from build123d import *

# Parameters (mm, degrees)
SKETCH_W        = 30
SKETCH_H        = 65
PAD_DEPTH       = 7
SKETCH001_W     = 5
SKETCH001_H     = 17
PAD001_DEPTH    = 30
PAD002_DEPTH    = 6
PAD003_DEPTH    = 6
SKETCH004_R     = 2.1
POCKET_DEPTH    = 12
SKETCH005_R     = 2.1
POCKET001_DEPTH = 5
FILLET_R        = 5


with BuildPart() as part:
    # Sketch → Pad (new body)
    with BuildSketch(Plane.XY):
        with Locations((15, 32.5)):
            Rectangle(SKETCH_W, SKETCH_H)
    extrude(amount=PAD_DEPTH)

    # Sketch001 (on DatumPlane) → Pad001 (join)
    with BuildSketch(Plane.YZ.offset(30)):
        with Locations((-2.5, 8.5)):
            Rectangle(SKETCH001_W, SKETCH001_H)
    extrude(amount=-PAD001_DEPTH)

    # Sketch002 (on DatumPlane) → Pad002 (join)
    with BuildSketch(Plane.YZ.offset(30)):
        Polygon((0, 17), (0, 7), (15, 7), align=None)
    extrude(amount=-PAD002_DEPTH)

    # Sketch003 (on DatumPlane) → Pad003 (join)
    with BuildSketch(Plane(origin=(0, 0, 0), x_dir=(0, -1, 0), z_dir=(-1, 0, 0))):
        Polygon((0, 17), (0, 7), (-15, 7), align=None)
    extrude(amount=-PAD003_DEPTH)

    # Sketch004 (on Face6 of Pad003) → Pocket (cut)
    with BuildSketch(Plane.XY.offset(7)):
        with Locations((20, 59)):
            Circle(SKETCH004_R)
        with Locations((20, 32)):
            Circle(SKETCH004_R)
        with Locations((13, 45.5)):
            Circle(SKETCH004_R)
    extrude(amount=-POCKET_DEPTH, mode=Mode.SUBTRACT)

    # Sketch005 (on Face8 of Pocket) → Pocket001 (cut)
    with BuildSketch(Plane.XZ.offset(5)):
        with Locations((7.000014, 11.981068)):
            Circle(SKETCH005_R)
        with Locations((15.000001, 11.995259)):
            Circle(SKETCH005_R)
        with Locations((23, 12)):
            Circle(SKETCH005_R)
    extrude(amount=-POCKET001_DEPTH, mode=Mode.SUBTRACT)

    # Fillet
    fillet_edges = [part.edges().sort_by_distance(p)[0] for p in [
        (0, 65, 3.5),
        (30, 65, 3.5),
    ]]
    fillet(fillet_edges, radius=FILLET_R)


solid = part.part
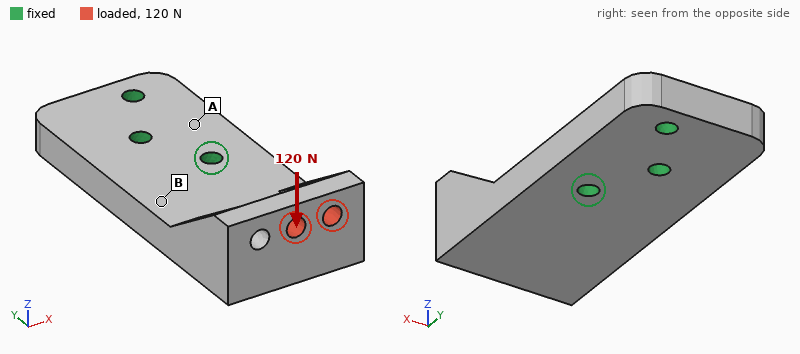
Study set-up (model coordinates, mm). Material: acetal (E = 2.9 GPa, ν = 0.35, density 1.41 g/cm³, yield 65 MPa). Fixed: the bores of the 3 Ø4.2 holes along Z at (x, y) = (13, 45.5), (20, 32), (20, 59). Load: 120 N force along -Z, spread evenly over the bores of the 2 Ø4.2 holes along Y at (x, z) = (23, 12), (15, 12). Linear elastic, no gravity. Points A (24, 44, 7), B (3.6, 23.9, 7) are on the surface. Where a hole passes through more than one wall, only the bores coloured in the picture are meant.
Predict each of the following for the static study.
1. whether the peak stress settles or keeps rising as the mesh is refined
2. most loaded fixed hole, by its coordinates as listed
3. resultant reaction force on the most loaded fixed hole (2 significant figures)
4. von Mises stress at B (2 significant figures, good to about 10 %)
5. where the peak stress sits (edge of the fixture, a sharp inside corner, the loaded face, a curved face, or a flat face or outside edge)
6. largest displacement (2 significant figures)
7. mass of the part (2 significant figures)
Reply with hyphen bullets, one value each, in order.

- keeps rising
- (20, 32)
- 220 N
- 10 MPa
- edge of the fixture
- 0.90 mm
- 23 g
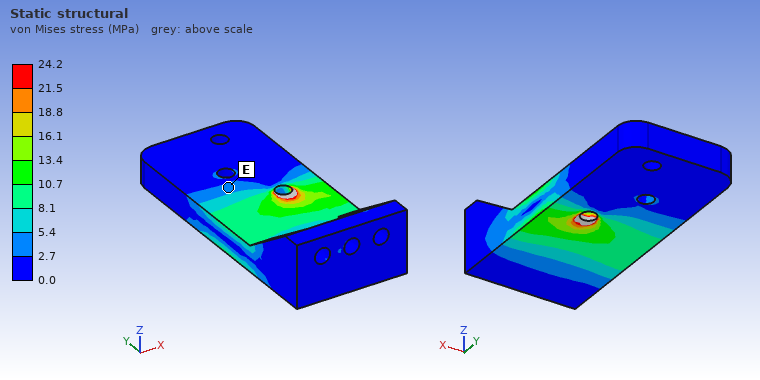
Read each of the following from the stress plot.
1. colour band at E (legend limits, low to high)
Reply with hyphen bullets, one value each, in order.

- 2.7 to 5.4 MPa
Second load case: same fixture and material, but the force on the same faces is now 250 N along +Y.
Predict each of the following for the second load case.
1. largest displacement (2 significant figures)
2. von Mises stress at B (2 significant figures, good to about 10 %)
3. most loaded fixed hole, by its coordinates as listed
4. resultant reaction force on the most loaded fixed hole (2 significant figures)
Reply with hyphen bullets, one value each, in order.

- 0.68 mm
- 7.7 MPa
- (20, 32)
- 190 N
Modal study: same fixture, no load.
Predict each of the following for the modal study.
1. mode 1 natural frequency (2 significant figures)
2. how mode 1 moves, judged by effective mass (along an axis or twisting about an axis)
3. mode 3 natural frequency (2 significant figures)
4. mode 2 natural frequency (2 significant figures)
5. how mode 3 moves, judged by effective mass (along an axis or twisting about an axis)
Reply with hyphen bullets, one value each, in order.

- 800 Hz
- along Z
- 2200 Hz
- 1700 Hz
- along X
